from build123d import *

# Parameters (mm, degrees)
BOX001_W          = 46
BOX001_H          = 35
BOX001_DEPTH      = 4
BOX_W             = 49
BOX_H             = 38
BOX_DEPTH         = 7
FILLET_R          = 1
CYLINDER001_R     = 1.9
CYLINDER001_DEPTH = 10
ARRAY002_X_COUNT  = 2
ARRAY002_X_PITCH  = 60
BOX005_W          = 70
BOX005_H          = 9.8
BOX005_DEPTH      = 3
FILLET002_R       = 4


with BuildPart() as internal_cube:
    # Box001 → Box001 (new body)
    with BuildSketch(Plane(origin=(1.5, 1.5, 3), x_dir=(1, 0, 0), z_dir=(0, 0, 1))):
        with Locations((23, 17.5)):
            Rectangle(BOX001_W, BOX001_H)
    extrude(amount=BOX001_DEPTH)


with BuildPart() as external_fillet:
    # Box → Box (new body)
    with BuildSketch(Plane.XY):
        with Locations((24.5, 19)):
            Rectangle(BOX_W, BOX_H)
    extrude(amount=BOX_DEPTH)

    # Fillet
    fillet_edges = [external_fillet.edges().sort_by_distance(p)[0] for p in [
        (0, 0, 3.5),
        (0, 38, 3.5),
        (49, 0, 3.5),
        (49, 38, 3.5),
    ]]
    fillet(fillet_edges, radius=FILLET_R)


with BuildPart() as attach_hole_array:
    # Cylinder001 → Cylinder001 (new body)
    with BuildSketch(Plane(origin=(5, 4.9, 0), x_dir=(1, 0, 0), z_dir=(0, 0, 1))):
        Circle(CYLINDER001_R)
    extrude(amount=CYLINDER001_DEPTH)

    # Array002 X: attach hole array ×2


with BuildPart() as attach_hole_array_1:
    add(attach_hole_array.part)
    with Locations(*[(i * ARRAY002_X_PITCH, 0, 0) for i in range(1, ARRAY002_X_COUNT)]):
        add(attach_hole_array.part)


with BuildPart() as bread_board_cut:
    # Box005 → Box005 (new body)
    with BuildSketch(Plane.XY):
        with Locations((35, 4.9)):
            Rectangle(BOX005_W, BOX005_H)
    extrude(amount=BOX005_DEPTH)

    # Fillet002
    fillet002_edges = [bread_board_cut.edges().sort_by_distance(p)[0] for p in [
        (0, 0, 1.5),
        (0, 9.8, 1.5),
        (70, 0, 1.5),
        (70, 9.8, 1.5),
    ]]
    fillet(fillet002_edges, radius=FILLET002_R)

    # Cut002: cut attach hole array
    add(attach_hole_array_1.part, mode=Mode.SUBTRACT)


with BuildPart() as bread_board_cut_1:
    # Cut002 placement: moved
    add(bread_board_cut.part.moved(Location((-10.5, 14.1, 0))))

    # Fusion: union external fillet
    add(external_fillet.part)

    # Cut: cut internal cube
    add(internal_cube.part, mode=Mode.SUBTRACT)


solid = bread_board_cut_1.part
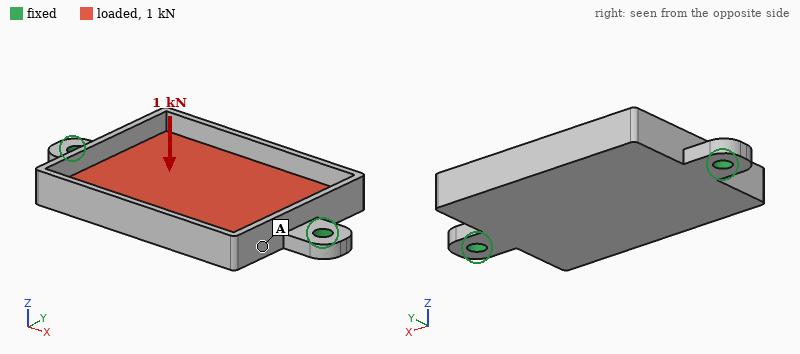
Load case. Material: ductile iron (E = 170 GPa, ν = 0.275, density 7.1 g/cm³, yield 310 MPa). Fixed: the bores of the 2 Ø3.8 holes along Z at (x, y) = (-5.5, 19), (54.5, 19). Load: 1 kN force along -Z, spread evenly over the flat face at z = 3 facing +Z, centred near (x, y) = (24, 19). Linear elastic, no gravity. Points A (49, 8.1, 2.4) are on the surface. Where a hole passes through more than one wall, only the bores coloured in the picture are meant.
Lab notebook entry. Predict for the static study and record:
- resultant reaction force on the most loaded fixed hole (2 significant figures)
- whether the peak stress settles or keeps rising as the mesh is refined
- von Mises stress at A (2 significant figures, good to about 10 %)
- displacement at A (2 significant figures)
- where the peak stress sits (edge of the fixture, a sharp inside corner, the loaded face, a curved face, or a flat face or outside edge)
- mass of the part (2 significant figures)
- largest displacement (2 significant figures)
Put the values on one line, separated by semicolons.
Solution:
500 N; keeps rising; 35 MPa; 16 µm; edge of the fixture; 50 g; 58 µm
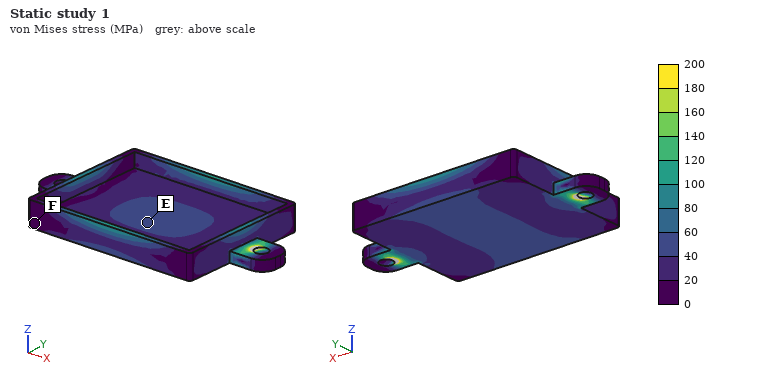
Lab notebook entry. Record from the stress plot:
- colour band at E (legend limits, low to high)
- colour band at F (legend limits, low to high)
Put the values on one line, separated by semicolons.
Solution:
40 to 60 MPa; 0 to 20 MPa
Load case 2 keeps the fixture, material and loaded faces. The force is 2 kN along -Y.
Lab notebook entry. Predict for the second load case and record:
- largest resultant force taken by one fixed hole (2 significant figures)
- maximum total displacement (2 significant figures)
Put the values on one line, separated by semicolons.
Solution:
1.0 kN; 42 µm
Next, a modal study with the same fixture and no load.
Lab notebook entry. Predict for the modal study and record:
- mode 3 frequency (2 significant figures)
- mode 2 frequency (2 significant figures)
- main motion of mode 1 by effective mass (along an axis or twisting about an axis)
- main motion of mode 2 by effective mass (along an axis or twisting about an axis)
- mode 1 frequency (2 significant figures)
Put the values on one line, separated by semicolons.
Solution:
6200 Hz; 3500 Hz; twisting about X; along Z; 2600 Hz
